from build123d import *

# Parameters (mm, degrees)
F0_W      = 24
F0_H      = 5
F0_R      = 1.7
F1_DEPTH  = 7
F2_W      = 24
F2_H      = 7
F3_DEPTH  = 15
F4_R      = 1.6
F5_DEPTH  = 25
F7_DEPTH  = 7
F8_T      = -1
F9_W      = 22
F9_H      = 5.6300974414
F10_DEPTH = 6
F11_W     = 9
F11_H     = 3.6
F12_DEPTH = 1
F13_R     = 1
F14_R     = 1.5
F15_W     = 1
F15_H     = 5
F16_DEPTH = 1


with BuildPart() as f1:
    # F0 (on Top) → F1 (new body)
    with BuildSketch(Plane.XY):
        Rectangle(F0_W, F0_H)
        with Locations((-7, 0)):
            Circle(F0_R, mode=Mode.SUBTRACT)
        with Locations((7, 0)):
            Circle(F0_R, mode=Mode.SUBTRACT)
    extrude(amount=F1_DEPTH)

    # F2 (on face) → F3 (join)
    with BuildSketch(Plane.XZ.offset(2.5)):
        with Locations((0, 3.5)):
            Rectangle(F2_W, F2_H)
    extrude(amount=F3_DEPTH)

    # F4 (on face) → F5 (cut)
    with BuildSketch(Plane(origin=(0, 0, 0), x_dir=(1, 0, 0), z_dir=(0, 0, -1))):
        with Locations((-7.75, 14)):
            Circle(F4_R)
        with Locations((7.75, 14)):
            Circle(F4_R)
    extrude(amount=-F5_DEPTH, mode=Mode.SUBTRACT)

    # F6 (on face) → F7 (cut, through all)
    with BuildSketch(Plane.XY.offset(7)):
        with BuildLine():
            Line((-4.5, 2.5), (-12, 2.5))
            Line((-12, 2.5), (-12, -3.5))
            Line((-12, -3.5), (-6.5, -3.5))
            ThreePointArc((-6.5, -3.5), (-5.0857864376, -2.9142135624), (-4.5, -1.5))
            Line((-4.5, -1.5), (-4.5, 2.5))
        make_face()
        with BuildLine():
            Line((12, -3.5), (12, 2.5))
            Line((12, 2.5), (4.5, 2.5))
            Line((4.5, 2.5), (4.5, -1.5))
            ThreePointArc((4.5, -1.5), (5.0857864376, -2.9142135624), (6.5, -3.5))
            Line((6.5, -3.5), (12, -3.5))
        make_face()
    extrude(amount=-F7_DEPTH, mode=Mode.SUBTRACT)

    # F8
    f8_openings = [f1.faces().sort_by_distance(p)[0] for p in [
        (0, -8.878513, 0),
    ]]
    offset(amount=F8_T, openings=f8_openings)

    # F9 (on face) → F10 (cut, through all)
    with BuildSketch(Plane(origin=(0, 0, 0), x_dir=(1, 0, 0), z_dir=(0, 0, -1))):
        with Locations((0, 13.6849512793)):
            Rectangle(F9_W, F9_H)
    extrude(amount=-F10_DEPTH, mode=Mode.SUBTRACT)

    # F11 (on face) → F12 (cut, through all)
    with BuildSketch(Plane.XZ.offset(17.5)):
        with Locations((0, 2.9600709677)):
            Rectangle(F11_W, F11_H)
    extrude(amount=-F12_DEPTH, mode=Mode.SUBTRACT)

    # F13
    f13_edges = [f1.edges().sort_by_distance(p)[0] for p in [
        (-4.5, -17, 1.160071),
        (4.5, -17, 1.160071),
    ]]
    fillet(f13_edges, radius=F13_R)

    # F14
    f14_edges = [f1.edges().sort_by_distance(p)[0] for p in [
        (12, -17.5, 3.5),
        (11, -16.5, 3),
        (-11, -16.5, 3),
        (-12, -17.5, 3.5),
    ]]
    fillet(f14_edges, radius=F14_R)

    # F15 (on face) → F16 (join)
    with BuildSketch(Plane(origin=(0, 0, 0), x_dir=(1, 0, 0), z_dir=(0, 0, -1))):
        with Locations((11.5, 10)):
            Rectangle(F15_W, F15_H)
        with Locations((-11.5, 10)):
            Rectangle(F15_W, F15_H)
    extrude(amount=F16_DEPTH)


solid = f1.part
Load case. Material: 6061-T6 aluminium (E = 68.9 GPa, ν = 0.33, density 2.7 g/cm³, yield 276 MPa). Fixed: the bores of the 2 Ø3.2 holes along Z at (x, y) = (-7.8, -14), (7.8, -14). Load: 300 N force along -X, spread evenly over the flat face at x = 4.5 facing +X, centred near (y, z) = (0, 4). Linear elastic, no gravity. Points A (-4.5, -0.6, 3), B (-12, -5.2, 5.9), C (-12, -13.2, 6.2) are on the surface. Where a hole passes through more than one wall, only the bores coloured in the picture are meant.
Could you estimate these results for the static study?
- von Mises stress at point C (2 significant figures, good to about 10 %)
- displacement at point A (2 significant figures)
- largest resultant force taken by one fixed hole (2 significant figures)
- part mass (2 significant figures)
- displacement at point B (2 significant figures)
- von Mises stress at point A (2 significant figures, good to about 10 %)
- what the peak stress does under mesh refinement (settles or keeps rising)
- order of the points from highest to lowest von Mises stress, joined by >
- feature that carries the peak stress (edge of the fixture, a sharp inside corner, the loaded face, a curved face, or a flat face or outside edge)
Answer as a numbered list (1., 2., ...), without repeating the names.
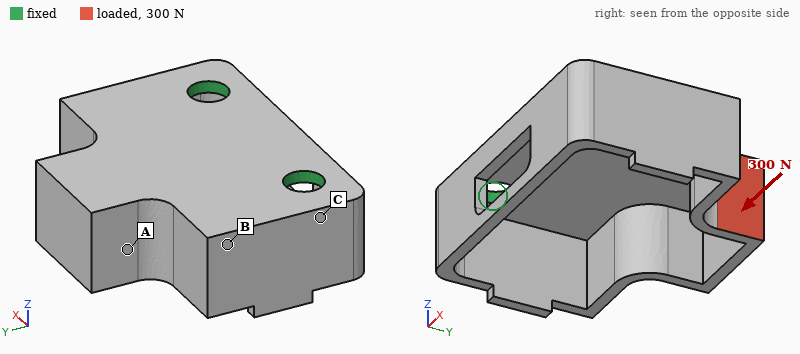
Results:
1. 38 MPa
2. 53 µm
3. 290 N
4. 2.3 g
5. 35 µm
6. 68 MPa
7. keeps rising
8. A > C > B
9. edge of the fixture
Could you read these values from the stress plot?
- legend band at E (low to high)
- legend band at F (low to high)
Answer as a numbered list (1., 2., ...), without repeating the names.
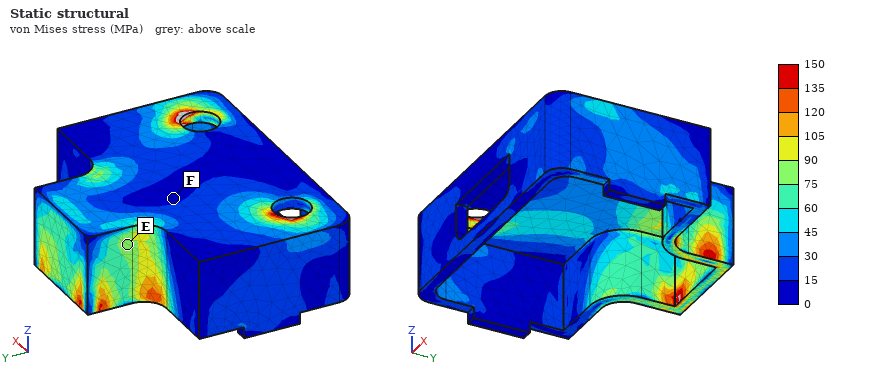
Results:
1. 75 to 90 MPa
2. 0 to 15 MPa
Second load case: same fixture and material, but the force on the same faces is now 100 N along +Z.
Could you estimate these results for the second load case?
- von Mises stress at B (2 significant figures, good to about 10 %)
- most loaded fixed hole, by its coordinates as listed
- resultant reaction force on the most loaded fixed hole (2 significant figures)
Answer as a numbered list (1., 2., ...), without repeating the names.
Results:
1. 40 MPa
2. (7.8, -14)
3. 75 N
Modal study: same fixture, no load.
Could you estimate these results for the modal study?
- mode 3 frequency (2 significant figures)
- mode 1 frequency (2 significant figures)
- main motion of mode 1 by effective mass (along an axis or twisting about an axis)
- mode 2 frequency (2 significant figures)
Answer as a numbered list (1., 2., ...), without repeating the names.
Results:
1. 11 kHz
2. 4400 Hz
3. along Z
4. 9100 Hz
